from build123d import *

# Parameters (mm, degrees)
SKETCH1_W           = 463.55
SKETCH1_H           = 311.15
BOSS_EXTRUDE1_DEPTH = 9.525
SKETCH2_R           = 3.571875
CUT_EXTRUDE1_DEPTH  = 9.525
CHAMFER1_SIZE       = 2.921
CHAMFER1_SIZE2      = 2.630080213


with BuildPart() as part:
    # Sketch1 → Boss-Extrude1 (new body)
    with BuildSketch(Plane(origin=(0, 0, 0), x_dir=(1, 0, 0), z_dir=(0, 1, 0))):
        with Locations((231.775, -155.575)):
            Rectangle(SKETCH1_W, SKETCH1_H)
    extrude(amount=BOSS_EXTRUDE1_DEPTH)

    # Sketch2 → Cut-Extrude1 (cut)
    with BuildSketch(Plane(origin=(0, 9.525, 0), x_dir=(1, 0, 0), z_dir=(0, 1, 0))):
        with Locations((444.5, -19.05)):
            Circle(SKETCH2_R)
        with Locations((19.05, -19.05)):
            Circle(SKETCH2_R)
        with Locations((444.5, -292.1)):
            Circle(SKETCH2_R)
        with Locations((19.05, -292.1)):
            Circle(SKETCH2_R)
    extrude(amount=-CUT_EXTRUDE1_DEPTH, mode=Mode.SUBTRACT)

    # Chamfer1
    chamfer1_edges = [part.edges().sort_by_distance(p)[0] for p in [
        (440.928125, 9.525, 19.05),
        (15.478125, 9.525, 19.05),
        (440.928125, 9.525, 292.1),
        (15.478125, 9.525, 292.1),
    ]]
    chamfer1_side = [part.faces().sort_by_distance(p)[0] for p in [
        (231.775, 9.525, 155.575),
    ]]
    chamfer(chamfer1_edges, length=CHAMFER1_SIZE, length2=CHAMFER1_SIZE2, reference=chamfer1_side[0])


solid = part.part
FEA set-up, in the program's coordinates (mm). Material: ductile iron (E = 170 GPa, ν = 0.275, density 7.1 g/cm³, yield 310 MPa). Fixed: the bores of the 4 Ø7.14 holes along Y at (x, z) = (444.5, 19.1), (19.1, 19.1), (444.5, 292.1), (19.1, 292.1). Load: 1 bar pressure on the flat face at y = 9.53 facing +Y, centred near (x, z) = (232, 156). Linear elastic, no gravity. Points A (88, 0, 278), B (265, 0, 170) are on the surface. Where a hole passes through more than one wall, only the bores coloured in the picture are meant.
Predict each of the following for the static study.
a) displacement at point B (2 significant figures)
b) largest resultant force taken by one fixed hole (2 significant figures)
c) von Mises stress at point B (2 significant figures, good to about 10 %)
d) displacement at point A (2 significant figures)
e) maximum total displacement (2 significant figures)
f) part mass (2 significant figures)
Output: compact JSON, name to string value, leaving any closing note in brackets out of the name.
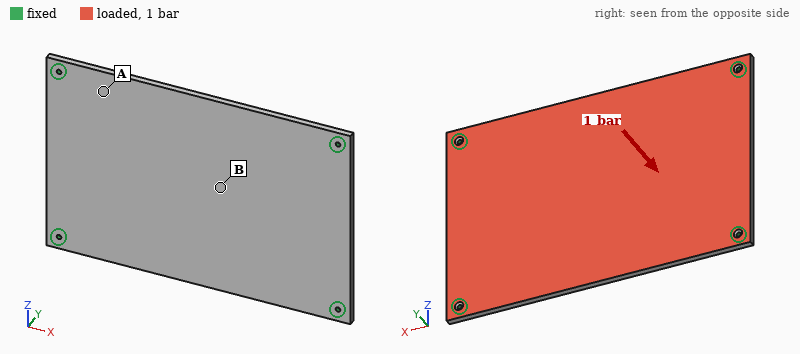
{"displacement at point B": "1.4 mm", "largest resultant force taken by one fixed hole": "4.4 kN", "von Mises stress at point B": "57 MPa", "displacement at point A": "0.53 mm", "maximum total displacement": "1.4 mm", "part mass": "9.7 kg"}
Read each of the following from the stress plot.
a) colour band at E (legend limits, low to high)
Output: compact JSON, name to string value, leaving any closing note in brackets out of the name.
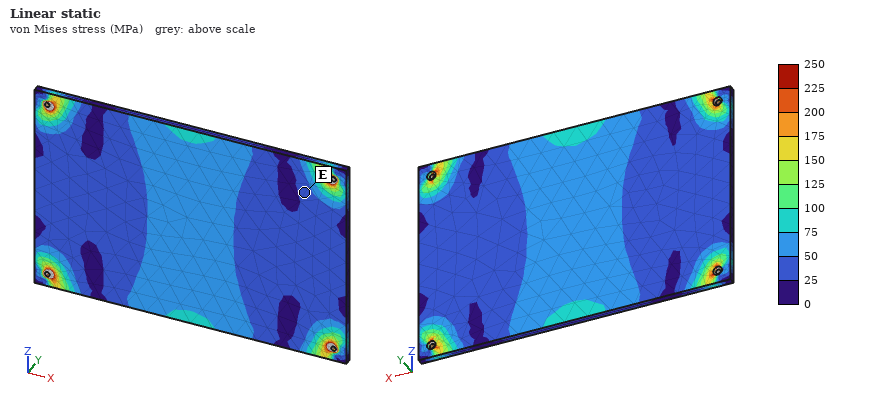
{"colour band at E": "25 to 50 MPa"}
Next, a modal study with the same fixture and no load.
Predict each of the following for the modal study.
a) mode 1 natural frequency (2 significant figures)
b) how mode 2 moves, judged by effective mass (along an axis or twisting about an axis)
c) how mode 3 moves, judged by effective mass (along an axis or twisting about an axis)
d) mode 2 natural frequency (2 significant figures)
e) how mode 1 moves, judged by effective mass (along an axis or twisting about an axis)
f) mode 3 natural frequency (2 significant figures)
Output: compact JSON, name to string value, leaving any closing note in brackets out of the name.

{"mode 1 natural frequency": "190 Hz", "how mode 2 moves, judged by effective mass": "twisting about X", "how mode 3 moves, judged by effective mass": "twisting about Z", "mode 2 natural frequency": "330 Hz", "how mode 1 moves, judged by effective mass": "along Y", "mode 3 natural frequency": "470 Hz"}
